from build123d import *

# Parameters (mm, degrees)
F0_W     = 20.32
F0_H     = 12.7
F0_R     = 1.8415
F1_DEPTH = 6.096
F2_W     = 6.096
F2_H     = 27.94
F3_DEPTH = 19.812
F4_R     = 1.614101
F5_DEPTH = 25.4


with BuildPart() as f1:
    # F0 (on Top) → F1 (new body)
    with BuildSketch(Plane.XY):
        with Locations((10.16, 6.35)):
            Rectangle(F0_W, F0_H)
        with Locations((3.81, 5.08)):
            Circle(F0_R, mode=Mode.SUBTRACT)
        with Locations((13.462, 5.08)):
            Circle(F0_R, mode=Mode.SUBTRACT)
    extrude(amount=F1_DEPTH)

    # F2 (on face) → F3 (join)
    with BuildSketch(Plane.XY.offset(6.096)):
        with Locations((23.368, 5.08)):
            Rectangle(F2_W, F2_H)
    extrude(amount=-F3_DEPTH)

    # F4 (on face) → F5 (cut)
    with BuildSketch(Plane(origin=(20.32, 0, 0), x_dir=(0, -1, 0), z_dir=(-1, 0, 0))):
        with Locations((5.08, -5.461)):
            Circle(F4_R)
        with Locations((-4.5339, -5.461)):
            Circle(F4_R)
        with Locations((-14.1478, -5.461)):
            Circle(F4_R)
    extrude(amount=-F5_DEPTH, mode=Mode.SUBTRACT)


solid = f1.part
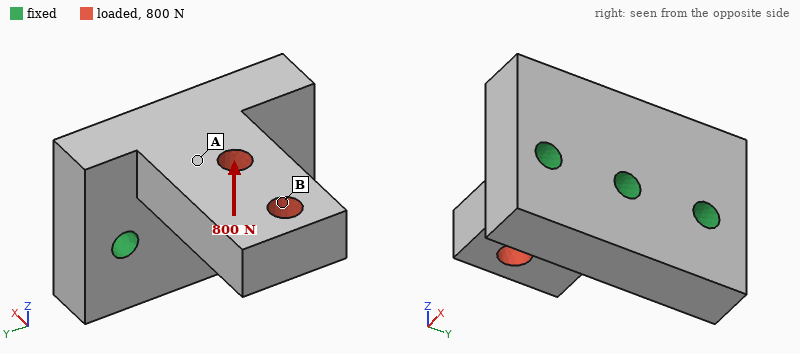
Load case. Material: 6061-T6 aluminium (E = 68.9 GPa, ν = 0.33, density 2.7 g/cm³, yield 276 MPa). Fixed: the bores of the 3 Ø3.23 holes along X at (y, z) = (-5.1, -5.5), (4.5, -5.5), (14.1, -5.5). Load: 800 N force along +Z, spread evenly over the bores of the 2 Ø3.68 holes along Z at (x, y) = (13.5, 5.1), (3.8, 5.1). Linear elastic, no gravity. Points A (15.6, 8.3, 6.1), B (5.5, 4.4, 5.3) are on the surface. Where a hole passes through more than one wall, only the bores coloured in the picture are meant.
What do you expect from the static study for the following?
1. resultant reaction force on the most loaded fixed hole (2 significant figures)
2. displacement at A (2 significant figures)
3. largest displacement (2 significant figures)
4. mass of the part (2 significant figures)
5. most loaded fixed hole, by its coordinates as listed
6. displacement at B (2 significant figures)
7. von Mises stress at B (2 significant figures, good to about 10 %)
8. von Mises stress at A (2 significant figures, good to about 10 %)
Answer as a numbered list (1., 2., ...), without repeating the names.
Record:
1. 590 N
2. 0.047 mm
3. 0.17 mm
4. 13 g
5. (4.5, -5.5)
6. 0.12 mm
7. 17 MPa
8. 88 MPa
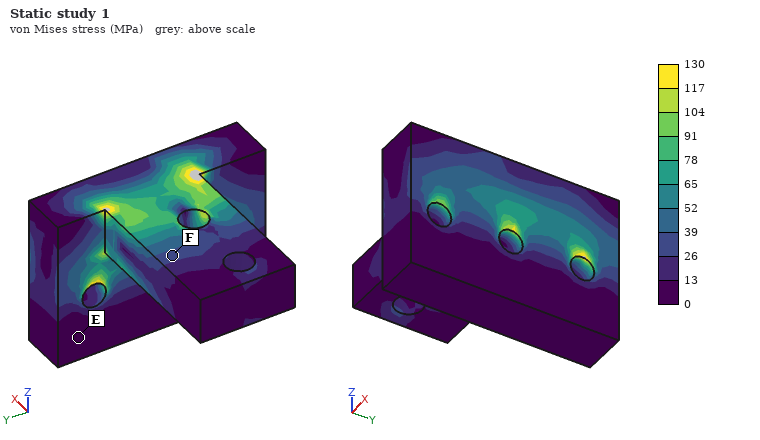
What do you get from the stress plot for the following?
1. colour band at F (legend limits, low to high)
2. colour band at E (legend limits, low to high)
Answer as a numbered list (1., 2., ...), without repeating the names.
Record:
1. 26 to 39 MPa
2. 0 to 13 MPa
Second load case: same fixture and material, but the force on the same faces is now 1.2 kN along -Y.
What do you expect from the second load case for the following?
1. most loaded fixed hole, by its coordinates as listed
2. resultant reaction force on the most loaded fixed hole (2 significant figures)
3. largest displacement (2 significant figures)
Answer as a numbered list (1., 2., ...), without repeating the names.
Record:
1. (14.1, -5.5)
2. 1.2 kN
3. 81 µm
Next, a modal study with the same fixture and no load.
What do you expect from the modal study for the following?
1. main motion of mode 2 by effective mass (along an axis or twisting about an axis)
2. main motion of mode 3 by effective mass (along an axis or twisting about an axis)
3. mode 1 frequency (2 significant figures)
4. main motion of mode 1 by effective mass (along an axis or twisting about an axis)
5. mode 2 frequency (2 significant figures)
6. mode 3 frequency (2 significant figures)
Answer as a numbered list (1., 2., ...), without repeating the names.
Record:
1. along Y
2. along X
3. 7500 Hz
4. along Z
5. 13 kHz
6. 24 kHz
